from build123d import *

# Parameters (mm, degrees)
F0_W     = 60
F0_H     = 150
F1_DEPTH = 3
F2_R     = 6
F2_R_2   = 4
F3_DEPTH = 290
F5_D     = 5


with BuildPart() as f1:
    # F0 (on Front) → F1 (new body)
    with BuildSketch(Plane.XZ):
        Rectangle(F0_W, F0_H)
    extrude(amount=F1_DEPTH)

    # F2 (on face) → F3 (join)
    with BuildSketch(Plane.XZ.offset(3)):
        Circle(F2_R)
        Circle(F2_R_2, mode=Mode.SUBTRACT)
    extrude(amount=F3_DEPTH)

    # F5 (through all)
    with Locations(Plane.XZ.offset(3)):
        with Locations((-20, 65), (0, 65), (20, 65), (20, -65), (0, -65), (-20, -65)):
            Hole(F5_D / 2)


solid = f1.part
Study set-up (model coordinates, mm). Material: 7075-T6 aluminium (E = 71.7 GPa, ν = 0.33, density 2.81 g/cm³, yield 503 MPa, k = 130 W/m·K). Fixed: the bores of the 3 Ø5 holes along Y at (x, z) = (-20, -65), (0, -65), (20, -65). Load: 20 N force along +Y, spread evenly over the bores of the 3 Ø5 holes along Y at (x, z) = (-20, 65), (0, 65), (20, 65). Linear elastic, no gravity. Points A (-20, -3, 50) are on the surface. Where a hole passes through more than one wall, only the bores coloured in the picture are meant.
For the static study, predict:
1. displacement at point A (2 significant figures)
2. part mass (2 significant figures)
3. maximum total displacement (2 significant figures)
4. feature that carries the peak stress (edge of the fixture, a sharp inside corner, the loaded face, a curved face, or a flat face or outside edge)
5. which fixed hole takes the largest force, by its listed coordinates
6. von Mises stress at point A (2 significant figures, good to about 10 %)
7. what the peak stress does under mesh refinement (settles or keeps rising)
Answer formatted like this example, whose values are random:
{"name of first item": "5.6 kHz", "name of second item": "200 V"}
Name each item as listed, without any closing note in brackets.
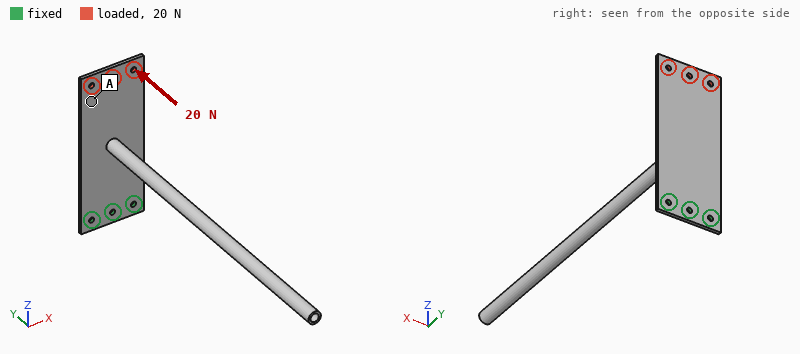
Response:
{"displacement at point A": "1.2 mm", "part mass": "130 g", "maximum total displacement": "3.6 mm", "feature that carries the peak stress": "edge of the fixture", "which fixed hole takes the largest force, by its listed coordinates": "(0, -65)", "von Mises stress at point A": "3.7 MPa", "what the peak stress does under mesh refinement": "keeps rising"}
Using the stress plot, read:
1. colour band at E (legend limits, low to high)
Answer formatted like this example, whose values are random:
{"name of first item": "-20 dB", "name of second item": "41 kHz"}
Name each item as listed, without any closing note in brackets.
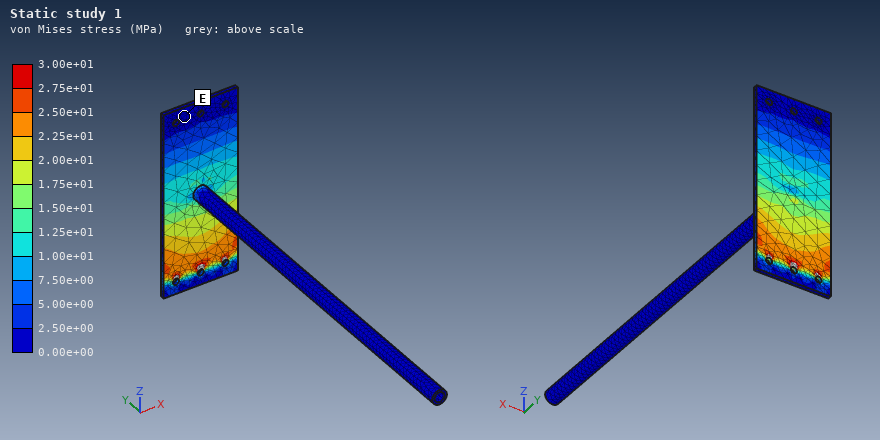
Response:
{"colour band at E": "0.00e+00 to 2.50e+00 MPa"}
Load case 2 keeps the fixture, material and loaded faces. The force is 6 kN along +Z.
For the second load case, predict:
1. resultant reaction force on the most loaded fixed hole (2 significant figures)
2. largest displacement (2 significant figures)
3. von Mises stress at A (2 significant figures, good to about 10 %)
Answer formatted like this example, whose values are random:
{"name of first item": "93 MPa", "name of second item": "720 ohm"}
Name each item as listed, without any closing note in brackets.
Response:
{"resultant reaction force on the most loaded fixed hole": "2.1 kN", "largest displacement": "68 µm", "von Mises stress at A": "34 MPa"}
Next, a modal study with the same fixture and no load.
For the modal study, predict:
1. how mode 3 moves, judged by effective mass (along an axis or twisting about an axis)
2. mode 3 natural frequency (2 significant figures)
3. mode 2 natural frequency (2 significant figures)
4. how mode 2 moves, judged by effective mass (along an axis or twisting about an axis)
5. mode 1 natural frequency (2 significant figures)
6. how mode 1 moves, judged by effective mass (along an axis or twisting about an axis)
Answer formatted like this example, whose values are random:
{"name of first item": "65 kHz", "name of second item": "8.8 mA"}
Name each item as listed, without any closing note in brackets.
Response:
{"how mode 3 moves, judged by effective mass": "along Y", "mode 3 natural frequency": "230 Hz", "mode 2 natural frequency": "62 Hz", "how mode 2 moves, judged by effective mass": "along X", "mode 1 natural frequency": "45 Hz", "how mode 1 moves, judged by effective mass": "along Z"}
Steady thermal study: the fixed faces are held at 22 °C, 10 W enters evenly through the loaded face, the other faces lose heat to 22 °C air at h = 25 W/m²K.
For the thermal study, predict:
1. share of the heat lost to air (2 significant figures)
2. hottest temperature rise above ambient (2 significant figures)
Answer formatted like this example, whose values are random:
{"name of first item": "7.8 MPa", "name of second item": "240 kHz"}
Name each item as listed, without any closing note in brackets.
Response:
{"share of the heat lost to air": "68 %", "hottest temperature rise above ambient": "30 K"}
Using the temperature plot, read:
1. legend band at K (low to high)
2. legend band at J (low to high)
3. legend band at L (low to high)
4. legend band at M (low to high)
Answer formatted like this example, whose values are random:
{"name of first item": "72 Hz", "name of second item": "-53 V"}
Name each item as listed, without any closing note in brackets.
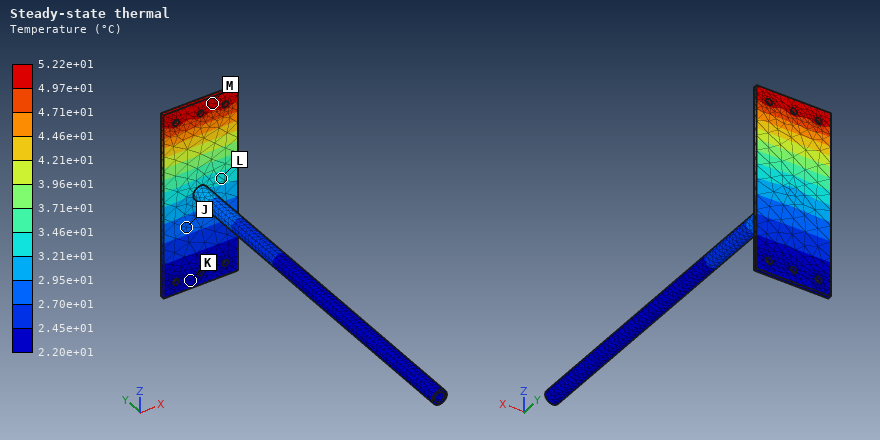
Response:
{"legend band at K": "2.20e+01 to 2.45e+01 °C", "legend band at J": "2.70e+01 to 2.95e+01 °C", "legend band at L": "3.21e+01 to 3.46e+01 °C", "legend band at M": "4.97e+01 to 5.22e+01 °C"}
